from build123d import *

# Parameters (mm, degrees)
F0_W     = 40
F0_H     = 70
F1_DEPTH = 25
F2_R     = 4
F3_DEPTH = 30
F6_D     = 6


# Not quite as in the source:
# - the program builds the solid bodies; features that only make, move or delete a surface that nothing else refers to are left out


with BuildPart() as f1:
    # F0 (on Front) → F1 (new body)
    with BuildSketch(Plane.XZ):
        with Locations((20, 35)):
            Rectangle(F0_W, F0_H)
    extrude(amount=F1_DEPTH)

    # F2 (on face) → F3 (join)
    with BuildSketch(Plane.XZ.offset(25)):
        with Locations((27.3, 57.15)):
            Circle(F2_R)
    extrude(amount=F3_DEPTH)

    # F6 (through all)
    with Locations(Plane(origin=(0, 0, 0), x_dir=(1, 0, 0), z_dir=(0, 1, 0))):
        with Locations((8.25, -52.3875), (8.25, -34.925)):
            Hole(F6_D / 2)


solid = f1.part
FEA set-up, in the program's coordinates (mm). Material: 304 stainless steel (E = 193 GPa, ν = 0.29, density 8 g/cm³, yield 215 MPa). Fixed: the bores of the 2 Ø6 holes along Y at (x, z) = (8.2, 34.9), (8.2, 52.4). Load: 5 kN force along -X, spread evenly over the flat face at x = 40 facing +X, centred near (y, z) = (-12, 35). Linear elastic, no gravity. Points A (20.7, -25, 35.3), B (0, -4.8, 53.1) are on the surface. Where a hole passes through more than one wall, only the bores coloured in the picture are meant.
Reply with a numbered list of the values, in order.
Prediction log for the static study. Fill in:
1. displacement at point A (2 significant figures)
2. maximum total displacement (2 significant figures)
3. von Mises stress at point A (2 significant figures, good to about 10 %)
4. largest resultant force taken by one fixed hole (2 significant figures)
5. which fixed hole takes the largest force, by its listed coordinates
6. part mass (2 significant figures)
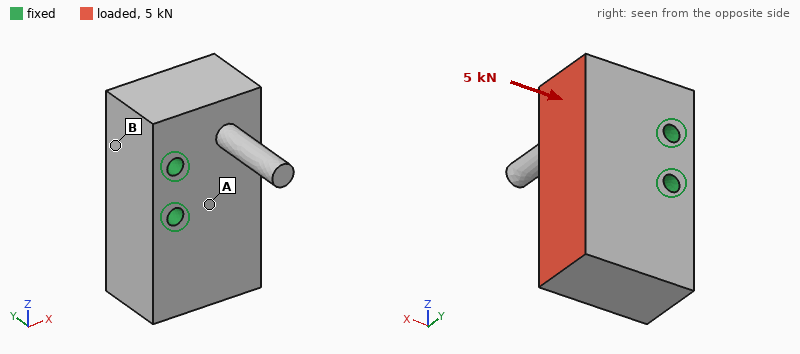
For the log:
1. 0.65 µm
2. 3.6 µm
3. 6.7 MPa
4. 4.3 kN
5. (8.2, 34.9)
6. 560 g
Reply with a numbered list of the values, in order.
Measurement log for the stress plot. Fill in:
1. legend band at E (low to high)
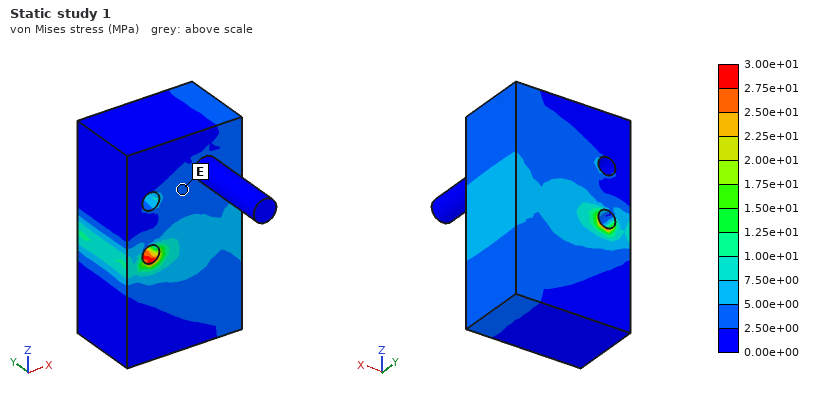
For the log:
1. 2.50e+00 to 5.00e+00 MPa
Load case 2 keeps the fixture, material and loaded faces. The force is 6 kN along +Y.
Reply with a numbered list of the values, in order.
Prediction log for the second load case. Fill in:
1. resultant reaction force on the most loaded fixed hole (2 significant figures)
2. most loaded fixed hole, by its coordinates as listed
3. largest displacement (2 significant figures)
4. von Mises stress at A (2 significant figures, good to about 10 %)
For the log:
1. 3.9 kN
2. (8.2, 34.9)
3. 14 µm
4. 24 MPa
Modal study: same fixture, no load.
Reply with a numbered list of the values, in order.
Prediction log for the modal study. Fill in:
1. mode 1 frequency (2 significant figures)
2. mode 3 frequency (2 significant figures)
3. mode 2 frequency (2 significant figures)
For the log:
1. 5200 Hz
2. 8100 Hz
3. 5200 Hz
